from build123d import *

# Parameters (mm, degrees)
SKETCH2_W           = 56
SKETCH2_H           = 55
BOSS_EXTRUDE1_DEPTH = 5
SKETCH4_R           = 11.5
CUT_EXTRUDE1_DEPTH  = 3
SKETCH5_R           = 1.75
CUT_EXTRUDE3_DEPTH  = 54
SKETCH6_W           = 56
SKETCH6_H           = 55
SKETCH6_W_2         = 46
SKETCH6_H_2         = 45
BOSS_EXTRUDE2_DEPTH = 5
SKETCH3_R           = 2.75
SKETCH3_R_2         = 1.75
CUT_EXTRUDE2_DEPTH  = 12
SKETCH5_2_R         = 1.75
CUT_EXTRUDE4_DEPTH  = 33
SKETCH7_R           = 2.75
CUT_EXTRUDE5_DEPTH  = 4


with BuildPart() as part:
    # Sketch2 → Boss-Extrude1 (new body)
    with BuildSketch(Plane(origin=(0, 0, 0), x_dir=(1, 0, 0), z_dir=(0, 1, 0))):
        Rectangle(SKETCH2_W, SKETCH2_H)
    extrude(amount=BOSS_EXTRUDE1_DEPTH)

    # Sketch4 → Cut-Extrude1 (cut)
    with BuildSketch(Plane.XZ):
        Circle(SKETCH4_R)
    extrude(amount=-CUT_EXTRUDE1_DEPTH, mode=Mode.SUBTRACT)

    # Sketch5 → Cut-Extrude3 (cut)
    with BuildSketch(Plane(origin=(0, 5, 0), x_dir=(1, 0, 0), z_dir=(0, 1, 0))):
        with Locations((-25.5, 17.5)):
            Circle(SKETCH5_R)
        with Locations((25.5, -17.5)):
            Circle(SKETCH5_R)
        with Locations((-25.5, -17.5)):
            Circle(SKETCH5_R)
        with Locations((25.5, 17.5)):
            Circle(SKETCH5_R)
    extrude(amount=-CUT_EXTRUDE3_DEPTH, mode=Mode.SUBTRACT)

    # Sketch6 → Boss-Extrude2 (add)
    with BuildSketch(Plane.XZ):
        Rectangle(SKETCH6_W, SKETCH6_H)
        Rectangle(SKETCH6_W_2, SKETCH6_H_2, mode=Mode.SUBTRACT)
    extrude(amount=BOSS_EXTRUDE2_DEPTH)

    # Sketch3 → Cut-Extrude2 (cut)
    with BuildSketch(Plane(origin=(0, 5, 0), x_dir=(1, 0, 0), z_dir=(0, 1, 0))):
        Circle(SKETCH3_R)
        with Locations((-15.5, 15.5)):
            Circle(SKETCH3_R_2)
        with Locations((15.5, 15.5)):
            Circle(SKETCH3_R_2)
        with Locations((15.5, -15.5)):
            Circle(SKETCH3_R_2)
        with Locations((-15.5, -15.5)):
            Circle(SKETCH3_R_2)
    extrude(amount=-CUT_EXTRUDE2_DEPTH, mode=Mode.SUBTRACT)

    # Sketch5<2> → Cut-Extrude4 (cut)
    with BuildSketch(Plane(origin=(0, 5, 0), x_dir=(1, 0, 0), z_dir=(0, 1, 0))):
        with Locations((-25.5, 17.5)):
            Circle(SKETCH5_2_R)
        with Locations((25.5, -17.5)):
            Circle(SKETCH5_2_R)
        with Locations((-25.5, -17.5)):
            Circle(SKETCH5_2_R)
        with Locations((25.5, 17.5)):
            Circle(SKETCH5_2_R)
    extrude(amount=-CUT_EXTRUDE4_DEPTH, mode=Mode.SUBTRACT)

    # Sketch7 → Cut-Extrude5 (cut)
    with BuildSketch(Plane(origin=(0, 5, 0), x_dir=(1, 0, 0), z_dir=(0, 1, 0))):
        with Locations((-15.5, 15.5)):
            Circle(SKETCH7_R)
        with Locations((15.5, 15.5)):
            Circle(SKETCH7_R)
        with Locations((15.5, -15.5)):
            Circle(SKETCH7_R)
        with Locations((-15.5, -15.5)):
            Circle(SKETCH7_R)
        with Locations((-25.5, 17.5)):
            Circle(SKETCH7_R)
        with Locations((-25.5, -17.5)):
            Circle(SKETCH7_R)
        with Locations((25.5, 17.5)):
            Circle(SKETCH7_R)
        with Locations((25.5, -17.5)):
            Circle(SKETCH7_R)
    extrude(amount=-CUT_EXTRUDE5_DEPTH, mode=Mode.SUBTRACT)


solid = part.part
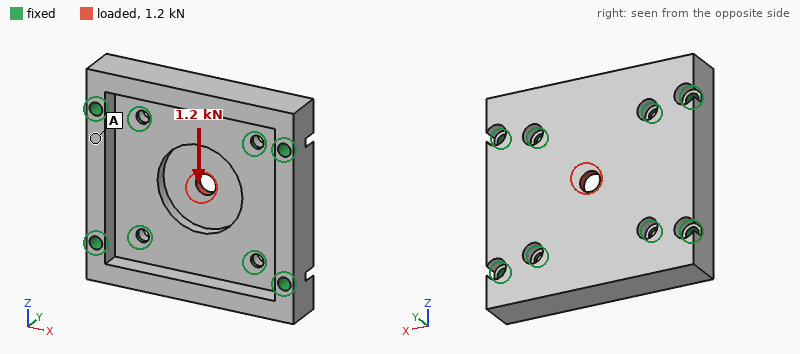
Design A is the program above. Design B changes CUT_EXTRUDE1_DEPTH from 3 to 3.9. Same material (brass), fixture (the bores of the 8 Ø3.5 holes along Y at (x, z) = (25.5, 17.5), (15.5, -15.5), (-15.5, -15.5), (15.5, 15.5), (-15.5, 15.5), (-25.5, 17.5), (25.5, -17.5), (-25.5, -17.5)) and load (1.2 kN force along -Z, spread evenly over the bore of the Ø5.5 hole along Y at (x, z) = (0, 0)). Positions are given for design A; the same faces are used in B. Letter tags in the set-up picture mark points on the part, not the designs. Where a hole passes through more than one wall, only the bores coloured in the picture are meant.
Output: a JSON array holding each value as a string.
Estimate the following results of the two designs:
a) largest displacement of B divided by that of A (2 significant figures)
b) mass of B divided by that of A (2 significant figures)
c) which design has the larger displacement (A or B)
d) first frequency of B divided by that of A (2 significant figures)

["1.6", "0.98", "B", "1.00"]
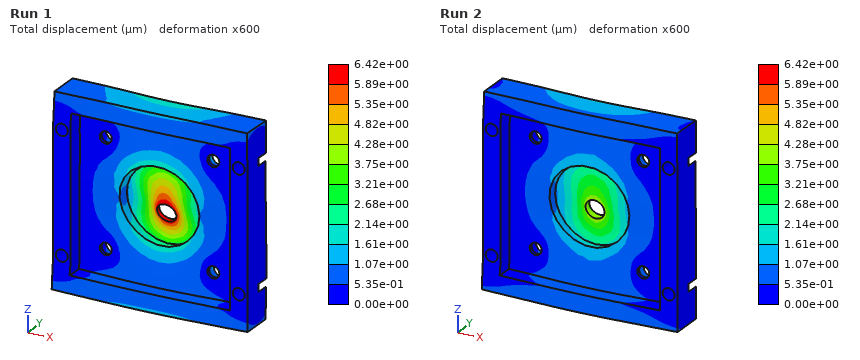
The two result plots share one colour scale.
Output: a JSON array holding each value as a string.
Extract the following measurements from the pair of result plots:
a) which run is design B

["Run 1"]
